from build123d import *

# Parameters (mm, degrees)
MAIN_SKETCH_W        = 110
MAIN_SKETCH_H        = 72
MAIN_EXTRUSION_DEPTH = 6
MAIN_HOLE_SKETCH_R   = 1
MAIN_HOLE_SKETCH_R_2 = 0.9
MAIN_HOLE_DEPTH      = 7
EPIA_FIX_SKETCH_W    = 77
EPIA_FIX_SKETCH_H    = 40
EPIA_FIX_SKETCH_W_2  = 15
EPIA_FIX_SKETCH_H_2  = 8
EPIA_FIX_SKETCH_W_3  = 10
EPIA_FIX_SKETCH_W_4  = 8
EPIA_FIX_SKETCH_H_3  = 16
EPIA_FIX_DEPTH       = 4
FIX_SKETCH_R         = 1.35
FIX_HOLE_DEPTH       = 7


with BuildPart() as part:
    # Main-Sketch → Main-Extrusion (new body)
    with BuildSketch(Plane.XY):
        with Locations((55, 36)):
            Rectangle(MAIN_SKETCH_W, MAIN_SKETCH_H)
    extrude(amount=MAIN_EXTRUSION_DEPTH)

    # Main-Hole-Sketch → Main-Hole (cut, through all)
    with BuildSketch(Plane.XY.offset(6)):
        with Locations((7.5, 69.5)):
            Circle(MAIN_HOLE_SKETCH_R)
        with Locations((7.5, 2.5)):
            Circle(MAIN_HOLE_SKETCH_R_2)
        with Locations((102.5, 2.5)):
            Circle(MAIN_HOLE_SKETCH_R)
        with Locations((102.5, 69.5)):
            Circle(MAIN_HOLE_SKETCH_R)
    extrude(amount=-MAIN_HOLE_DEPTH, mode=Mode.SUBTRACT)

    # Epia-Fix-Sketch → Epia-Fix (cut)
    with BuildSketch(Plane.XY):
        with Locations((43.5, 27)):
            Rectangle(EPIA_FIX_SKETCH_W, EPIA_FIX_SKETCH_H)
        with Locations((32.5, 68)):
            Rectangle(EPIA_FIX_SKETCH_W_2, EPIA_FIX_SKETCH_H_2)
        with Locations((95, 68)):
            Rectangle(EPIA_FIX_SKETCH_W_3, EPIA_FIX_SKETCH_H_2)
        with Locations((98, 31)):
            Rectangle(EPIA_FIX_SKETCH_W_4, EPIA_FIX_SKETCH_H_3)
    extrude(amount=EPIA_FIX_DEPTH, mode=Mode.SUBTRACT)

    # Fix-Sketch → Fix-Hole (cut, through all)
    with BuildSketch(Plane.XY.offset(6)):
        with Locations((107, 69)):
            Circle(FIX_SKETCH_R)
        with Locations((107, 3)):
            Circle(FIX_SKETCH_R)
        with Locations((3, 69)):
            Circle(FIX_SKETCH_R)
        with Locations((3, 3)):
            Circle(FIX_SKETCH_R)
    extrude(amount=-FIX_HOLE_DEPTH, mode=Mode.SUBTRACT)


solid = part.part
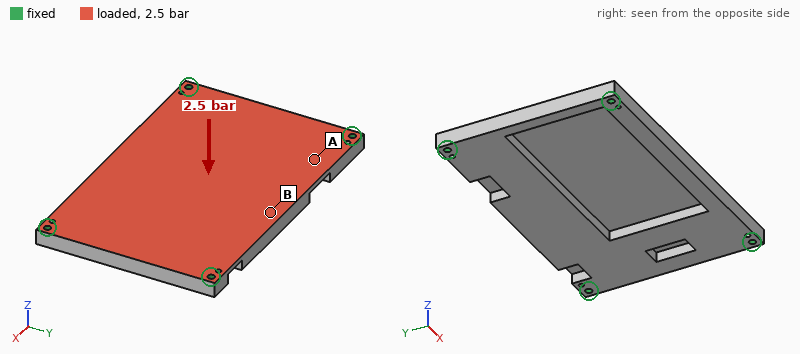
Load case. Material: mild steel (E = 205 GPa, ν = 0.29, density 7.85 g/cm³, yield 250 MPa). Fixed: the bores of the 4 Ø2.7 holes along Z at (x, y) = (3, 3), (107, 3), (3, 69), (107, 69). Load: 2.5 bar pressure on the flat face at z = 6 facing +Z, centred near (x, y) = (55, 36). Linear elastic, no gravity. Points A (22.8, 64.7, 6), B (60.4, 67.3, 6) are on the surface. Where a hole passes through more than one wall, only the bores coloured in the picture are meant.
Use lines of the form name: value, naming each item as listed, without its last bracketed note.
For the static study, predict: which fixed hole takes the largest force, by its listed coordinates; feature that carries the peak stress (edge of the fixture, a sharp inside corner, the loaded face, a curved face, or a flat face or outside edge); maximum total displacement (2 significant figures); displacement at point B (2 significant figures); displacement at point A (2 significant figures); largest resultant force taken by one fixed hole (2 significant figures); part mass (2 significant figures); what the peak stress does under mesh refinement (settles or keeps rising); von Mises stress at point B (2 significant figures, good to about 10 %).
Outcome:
which fixed hole takes the largest force, by its listed coordinates: (107, 3)
feature that carries the peak stress: edge of the fixture
maximum total displacement: 89 µm
displacement at point B: 55 µm
displacement at point A: 28 µm
largest resultant force taken by one fixed hole: 880 N
part mass: 260 g
what the peak stress does under mesh refinement: keeps rising
von Mises stress at point B: 34 MPa
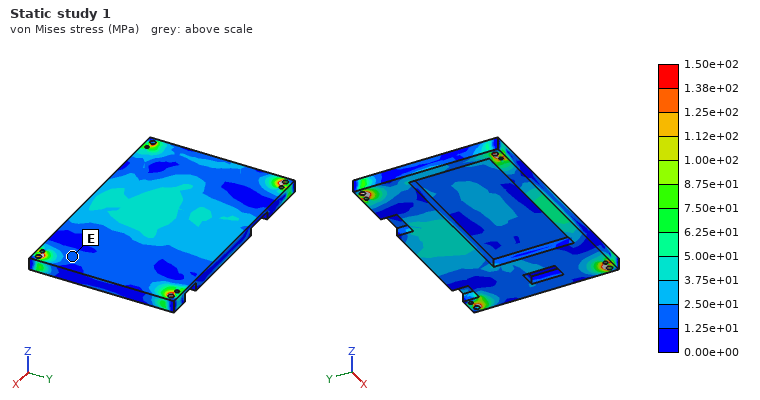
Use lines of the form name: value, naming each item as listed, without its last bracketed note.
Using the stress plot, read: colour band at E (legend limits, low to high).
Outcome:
colour band at E: 1.25e+01 to 2.50e+01 MPa
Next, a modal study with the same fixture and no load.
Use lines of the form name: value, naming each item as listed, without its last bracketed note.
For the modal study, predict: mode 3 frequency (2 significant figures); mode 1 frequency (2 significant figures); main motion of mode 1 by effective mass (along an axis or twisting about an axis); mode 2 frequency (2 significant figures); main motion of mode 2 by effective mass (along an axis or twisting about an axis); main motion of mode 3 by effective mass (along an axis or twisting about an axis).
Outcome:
mode 3 frequency: 4500 Hz
mode 1 frequency: 2000 Hz
main motion of mode 1 by effective mass: along Z
mode 2 frequency: 3100 Hz
main motion of mode 2 by effective mass: twisting about X
main motion of mode 3 by effective mass: twisting about Y
